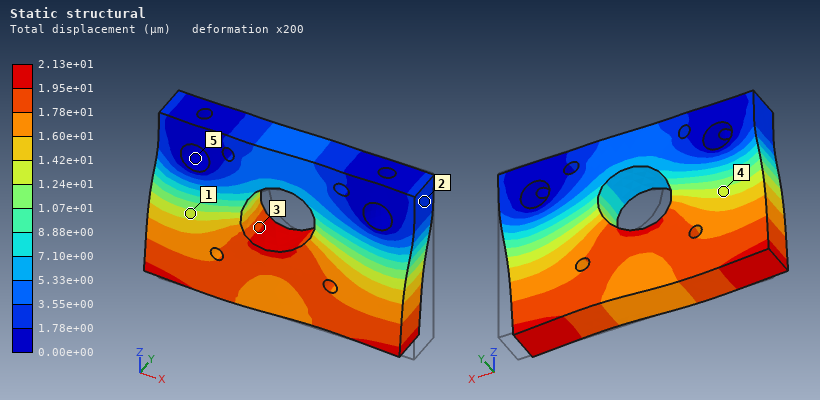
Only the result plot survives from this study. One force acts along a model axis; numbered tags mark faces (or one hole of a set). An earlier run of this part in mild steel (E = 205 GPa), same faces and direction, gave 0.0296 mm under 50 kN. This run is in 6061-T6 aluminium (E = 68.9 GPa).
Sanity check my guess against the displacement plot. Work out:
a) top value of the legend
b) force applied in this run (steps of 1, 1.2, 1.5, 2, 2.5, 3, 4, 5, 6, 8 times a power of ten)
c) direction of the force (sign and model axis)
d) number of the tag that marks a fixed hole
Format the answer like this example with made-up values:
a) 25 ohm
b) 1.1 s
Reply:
a) 2.13e+01 µm
b) 12 kN
c) -X
d) 5
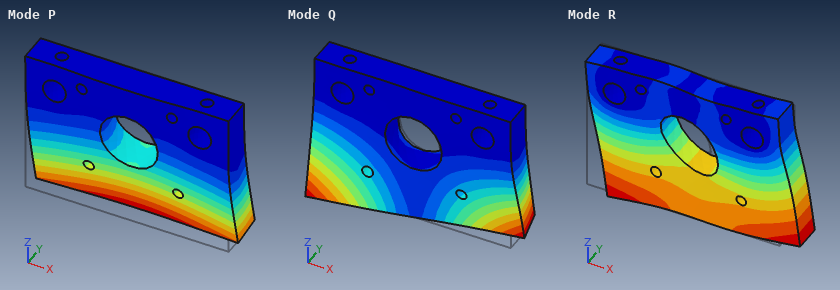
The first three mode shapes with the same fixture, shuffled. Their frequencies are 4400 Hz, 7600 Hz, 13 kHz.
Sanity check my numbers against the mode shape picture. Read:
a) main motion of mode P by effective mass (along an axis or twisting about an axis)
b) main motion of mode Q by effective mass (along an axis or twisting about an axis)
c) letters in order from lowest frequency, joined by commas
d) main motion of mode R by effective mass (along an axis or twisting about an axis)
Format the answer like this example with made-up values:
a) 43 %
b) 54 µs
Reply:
a) along Y
b) twisting about Z
c) P, Q, R
d) along X
